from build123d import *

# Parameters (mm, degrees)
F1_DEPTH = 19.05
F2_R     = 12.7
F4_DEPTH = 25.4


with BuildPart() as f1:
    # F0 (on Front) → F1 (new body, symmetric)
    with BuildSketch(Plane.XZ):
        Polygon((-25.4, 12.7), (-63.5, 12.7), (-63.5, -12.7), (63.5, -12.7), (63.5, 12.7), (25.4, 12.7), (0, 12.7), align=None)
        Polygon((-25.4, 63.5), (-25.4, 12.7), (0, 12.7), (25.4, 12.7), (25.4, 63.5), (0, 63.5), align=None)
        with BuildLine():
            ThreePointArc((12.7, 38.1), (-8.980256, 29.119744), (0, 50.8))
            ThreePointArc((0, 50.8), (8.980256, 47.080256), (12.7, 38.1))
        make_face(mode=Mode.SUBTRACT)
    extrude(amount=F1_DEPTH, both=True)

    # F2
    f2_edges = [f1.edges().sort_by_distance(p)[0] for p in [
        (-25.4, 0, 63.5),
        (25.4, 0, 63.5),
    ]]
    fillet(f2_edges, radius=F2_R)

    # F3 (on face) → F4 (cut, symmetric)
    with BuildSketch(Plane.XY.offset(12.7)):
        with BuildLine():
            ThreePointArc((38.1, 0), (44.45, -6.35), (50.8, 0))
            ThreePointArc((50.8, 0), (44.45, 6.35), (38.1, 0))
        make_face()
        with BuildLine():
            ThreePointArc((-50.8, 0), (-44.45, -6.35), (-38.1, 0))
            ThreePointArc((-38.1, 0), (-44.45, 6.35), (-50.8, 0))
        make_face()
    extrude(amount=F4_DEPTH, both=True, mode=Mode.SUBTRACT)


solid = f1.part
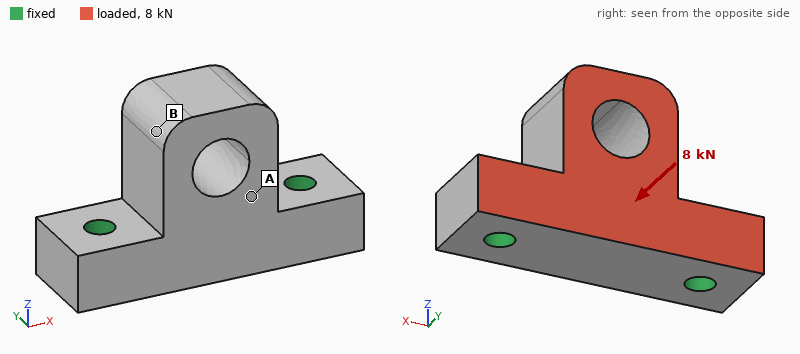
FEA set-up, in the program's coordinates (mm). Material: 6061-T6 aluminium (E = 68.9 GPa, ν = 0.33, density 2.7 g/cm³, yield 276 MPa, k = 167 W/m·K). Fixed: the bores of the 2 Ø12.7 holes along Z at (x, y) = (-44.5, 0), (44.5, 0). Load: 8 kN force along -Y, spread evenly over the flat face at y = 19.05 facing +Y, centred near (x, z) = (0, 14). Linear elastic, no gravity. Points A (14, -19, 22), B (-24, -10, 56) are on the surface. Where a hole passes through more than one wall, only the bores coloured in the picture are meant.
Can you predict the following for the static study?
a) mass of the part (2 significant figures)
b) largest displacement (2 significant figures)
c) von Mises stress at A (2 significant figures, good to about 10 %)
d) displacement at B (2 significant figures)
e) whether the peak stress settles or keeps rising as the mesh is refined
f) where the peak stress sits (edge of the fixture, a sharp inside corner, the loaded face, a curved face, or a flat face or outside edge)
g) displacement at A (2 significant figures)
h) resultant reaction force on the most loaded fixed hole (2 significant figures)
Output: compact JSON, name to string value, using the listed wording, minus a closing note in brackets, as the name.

{"mass of the part": "520 g", "largest displacement": "42 µm", "von Mises stress at A": "5.8 MPa", "displacement at B": "35 µm", "whether the peak stress settles or keeps rising as the mesh is refined": "keeps rising", "where the peak stress sits": "edge of the fixture", "displacement at A": "18 µm", "resultant reaction force on the most loaded fixed hole": "4.0 kN"}
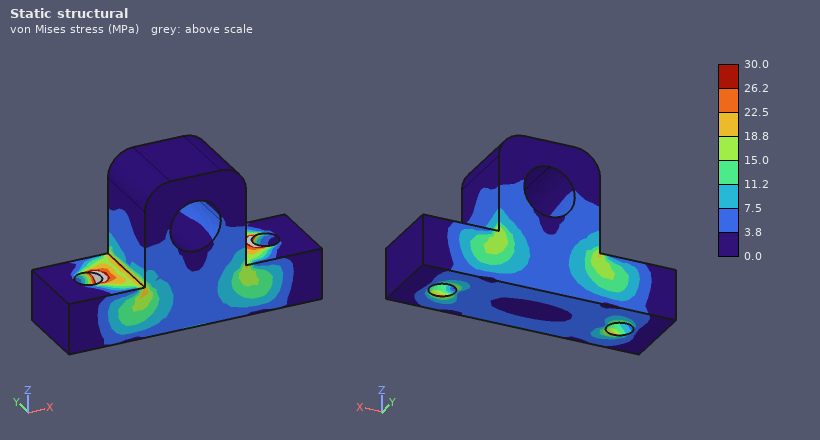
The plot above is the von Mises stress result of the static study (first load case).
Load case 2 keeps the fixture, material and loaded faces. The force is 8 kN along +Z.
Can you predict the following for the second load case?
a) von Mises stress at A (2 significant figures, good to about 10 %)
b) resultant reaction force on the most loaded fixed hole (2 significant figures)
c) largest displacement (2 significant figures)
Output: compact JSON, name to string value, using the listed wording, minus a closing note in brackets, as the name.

{"von Mises stress at A": "4.3 MPa", "resultant reaction force on the most loaded fixed hole": "4.1 kN", "largest displacement": "36 µm"}
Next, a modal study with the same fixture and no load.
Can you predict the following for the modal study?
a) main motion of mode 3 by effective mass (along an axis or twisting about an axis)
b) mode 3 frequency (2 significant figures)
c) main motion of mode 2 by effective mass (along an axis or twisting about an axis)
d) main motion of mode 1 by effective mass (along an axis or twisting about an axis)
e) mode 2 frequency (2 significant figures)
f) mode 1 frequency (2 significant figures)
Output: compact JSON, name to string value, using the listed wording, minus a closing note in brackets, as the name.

{"main motion of mode 3 by effective mass": "along Z", "mode 3 frequency": "9000 Hz", "main motion of mode 2 by effective mass": "along X", "main motion of mode 1 by effective mass": "along Y", "mode 2 frequency": "6300 Hz", "mode 1 frequency": "3600 Hz"}
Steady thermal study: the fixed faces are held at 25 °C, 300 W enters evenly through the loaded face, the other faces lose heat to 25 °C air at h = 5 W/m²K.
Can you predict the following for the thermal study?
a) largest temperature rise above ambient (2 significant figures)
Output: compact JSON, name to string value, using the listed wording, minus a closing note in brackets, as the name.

{"largest temperature rise above ambient": "36 K"}
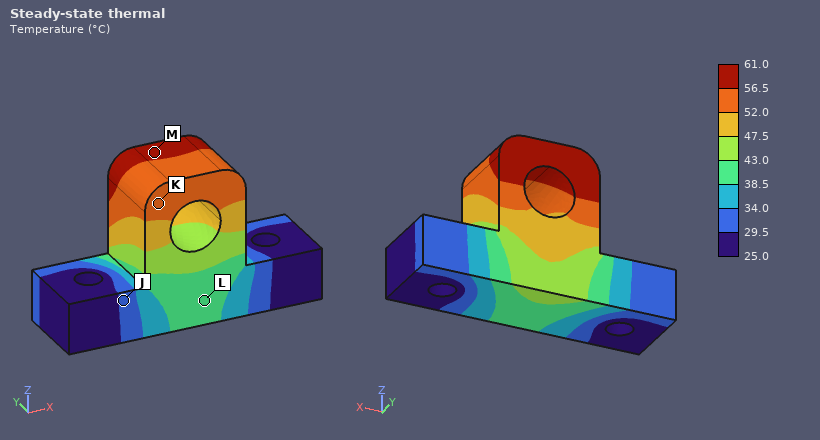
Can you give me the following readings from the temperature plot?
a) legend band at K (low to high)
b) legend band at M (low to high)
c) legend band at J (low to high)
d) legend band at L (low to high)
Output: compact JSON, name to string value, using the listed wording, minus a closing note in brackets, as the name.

{"legend band at K": "52.0 to 56.5 °C", "legend band at M": "56.5 to 61.0 °C", "legend band at J": "29.5 to 34.0 °C", "legend band at L": "38.5 to 43.0 °C"}
